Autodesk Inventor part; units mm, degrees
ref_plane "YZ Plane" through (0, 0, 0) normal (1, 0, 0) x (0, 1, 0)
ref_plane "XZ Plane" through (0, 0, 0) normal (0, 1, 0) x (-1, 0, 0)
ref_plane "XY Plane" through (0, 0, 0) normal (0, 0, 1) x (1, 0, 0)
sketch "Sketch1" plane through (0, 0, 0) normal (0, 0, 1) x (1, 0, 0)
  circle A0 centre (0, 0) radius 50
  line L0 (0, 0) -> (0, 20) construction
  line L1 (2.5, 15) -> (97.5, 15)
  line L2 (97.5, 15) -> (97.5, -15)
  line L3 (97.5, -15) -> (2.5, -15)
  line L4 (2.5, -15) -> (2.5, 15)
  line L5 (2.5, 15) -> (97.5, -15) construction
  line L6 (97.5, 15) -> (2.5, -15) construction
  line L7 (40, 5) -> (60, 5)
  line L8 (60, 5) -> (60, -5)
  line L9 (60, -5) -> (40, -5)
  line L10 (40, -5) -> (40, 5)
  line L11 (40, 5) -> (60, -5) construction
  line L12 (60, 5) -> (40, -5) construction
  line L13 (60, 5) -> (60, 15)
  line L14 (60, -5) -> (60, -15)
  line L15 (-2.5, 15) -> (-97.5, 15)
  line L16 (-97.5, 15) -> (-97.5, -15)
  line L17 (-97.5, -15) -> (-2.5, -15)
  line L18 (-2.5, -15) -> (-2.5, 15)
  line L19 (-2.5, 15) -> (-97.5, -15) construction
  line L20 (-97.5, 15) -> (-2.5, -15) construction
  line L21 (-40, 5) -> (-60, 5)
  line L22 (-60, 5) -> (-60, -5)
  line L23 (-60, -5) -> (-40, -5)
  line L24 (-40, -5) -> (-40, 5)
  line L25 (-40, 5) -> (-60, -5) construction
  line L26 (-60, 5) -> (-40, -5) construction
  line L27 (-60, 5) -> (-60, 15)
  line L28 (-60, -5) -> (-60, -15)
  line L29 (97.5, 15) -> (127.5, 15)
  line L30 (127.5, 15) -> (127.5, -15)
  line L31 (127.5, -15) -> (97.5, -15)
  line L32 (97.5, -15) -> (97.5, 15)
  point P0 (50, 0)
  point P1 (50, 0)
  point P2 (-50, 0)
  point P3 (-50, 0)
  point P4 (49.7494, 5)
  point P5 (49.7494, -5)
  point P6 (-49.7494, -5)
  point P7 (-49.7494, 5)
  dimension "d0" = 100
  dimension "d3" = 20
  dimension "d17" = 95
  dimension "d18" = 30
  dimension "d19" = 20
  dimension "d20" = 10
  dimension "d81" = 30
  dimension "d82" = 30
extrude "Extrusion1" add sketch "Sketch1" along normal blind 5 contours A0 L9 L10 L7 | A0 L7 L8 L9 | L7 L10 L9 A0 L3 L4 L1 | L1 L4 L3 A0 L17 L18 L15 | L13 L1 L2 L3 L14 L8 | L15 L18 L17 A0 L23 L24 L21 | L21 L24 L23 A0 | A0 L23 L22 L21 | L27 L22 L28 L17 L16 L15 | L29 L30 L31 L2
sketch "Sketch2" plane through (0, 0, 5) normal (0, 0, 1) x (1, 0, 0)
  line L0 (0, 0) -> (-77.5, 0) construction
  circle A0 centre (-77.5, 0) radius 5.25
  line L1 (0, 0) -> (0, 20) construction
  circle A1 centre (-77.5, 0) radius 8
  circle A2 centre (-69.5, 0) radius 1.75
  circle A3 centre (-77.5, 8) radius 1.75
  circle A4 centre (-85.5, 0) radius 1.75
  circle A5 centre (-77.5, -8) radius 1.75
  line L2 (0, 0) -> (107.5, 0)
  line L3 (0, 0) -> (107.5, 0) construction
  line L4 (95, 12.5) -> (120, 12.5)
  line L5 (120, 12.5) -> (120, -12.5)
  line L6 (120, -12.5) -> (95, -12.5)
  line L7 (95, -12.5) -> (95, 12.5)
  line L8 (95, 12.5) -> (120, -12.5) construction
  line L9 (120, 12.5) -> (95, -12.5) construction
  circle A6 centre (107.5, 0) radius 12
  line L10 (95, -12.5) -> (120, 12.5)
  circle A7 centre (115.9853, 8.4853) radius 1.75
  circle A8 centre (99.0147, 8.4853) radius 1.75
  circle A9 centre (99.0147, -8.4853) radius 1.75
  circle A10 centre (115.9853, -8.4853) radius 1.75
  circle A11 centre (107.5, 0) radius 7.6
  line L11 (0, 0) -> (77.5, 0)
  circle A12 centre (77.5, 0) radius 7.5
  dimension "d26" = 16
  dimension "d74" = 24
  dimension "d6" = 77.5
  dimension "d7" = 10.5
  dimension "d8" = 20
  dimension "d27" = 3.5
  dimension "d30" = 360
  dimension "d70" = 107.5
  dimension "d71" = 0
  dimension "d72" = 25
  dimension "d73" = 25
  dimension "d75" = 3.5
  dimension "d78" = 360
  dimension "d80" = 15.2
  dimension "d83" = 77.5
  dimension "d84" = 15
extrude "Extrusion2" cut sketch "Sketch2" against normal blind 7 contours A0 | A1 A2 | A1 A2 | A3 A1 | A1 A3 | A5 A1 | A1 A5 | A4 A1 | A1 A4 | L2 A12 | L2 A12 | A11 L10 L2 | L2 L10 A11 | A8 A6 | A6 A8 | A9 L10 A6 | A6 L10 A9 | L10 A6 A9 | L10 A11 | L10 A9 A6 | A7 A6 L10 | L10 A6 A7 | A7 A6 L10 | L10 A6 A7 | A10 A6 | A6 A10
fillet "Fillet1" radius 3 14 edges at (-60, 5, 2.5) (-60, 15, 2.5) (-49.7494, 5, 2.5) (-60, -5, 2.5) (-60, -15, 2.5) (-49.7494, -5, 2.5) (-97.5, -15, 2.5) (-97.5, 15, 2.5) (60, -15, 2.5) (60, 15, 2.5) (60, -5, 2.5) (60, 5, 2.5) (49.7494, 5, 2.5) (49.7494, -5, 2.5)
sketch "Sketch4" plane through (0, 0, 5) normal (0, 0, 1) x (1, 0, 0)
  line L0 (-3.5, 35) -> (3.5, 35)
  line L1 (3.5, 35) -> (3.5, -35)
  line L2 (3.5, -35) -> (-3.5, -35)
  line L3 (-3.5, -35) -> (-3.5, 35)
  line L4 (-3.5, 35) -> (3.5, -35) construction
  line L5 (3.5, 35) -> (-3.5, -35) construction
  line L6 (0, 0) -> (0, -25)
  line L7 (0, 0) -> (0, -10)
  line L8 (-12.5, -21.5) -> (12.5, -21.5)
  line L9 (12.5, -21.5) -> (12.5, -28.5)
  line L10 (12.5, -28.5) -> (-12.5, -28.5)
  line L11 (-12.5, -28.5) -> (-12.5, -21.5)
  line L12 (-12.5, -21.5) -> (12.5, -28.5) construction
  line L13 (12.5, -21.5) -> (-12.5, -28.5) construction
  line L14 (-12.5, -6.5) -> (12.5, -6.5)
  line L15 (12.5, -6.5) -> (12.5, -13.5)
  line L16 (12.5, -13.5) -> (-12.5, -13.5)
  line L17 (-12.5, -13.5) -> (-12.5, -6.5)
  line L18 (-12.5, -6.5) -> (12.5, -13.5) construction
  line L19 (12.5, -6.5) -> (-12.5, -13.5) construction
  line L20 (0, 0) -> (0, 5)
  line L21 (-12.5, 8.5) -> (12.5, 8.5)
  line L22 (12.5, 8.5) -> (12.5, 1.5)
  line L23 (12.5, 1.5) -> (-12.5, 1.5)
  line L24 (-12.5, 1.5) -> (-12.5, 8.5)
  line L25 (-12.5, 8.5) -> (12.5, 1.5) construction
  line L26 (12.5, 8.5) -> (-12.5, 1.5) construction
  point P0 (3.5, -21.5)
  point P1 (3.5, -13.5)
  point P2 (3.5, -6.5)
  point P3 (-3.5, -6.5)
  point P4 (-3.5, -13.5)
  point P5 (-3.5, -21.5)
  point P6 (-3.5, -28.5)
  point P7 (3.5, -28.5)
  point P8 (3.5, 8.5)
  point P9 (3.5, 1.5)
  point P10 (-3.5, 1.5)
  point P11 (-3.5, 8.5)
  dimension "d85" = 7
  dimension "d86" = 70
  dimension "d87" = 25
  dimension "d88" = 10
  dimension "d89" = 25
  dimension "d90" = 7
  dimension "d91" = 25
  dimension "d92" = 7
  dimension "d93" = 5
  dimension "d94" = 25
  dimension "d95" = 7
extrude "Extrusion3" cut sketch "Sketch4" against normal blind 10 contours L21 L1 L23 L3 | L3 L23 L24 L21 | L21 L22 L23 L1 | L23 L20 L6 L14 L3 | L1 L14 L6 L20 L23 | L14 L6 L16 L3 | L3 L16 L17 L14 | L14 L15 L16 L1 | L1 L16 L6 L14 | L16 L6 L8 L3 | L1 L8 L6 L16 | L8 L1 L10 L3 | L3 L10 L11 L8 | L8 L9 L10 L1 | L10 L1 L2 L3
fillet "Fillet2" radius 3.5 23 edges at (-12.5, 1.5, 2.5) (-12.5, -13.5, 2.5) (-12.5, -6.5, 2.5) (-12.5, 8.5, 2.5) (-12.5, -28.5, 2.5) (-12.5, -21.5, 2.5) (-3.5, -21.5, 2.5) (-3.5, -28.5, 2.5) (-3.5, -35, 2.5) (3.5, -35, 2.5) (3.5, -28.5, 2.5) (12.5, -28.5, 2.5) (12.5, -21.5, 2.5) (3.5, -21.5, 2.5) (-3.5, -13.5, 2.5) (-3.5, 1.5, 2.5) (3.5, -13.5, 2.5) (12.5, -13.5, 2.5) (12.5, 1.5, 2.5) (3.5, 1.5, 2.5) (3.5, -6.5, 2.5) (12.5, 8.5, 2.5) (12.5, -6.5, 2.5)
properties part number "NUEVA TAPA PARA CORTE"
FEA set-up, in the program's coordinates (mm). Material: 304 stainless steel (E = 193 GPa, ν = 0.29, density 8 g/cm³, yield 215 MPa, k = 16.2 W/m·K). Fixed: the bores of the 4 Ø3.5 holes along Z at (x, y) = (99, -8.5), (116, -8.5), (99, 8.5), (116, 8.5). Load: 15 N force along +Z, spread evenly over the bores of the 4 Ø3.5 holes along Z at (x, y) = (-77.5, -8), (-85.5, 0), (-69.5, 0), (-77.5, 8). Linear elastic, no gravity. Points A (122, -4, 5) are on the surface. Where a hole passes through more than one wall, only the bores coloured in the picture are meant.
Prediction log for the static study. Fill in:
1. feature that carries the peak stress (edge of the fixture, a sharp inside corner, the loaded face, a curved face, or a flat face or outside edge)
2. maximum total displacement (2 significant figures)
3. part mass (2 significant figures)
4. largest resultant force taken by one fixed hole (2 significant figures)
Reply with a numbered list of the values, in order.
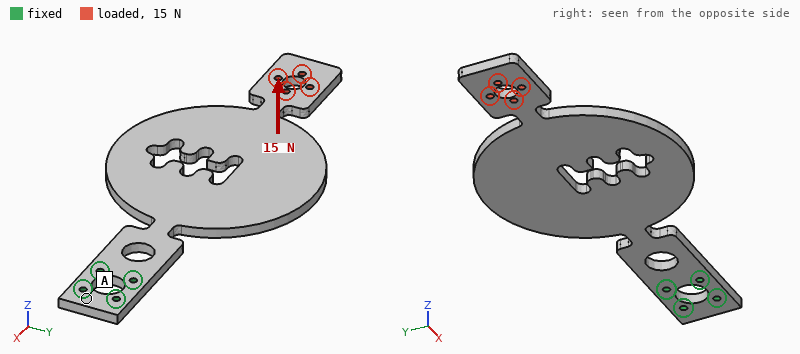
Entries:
1. a curved face
2. 0.74 mm
3. 400 g
4. 16 N
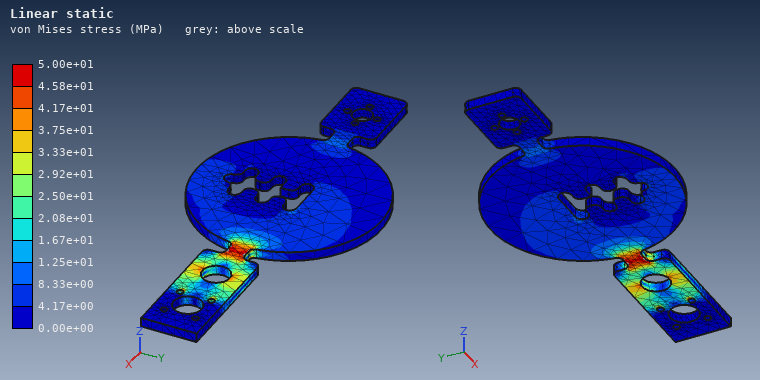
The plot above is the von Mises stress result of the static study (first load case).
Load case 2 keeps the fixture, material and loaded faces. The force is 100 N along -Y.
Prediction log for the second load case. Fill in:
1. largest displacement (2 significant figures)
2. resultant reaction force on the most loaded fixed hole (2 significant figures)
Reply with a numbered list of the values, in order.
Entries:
1. 0.45 mm
2. 790 N
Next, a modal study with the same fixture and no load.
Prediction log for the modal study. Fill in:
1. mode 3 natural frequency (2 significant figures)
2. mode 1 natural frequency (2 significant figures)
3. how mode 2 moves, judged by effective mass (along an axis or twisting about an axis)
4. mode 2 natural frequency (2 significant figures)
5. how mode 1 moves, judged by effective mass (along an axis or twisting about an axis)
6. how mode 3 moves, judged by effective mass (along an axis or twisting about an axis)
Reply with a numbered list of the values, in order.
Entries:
1. 300 Hz
2. 74 Hz
3. along Y
4. 240 Hz
5. along Z
6. twisting about X
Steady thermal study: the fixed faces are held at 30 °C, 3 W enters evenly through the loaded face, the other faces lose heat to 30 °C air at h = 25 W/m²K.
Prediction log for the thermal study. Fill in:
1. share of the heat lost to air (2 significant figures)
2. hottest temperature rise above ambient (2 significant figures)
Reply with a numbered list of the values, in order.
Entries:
1. 100 %
2. 35 K
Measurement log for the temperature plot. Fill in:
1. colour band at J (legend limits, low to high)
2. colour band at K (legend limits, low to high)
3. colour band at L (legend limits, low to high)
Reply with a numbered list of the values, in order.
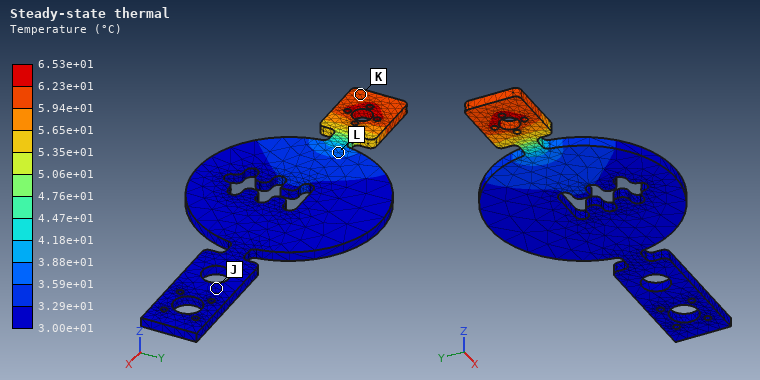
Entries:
1. 3.00e+01 to 3.29e+01 °C
2. 5.94e+01 to 6.23e+01 °C
3. 3.59e+01 to 3.88e+01 °C
